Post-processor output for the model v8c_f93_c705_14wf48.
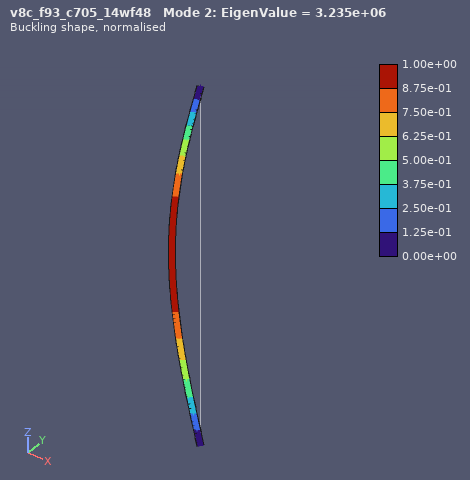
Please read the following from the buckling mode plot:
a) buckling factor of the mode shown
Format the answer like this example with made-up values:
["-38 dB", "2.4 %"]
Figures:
["3.235e+06"]
